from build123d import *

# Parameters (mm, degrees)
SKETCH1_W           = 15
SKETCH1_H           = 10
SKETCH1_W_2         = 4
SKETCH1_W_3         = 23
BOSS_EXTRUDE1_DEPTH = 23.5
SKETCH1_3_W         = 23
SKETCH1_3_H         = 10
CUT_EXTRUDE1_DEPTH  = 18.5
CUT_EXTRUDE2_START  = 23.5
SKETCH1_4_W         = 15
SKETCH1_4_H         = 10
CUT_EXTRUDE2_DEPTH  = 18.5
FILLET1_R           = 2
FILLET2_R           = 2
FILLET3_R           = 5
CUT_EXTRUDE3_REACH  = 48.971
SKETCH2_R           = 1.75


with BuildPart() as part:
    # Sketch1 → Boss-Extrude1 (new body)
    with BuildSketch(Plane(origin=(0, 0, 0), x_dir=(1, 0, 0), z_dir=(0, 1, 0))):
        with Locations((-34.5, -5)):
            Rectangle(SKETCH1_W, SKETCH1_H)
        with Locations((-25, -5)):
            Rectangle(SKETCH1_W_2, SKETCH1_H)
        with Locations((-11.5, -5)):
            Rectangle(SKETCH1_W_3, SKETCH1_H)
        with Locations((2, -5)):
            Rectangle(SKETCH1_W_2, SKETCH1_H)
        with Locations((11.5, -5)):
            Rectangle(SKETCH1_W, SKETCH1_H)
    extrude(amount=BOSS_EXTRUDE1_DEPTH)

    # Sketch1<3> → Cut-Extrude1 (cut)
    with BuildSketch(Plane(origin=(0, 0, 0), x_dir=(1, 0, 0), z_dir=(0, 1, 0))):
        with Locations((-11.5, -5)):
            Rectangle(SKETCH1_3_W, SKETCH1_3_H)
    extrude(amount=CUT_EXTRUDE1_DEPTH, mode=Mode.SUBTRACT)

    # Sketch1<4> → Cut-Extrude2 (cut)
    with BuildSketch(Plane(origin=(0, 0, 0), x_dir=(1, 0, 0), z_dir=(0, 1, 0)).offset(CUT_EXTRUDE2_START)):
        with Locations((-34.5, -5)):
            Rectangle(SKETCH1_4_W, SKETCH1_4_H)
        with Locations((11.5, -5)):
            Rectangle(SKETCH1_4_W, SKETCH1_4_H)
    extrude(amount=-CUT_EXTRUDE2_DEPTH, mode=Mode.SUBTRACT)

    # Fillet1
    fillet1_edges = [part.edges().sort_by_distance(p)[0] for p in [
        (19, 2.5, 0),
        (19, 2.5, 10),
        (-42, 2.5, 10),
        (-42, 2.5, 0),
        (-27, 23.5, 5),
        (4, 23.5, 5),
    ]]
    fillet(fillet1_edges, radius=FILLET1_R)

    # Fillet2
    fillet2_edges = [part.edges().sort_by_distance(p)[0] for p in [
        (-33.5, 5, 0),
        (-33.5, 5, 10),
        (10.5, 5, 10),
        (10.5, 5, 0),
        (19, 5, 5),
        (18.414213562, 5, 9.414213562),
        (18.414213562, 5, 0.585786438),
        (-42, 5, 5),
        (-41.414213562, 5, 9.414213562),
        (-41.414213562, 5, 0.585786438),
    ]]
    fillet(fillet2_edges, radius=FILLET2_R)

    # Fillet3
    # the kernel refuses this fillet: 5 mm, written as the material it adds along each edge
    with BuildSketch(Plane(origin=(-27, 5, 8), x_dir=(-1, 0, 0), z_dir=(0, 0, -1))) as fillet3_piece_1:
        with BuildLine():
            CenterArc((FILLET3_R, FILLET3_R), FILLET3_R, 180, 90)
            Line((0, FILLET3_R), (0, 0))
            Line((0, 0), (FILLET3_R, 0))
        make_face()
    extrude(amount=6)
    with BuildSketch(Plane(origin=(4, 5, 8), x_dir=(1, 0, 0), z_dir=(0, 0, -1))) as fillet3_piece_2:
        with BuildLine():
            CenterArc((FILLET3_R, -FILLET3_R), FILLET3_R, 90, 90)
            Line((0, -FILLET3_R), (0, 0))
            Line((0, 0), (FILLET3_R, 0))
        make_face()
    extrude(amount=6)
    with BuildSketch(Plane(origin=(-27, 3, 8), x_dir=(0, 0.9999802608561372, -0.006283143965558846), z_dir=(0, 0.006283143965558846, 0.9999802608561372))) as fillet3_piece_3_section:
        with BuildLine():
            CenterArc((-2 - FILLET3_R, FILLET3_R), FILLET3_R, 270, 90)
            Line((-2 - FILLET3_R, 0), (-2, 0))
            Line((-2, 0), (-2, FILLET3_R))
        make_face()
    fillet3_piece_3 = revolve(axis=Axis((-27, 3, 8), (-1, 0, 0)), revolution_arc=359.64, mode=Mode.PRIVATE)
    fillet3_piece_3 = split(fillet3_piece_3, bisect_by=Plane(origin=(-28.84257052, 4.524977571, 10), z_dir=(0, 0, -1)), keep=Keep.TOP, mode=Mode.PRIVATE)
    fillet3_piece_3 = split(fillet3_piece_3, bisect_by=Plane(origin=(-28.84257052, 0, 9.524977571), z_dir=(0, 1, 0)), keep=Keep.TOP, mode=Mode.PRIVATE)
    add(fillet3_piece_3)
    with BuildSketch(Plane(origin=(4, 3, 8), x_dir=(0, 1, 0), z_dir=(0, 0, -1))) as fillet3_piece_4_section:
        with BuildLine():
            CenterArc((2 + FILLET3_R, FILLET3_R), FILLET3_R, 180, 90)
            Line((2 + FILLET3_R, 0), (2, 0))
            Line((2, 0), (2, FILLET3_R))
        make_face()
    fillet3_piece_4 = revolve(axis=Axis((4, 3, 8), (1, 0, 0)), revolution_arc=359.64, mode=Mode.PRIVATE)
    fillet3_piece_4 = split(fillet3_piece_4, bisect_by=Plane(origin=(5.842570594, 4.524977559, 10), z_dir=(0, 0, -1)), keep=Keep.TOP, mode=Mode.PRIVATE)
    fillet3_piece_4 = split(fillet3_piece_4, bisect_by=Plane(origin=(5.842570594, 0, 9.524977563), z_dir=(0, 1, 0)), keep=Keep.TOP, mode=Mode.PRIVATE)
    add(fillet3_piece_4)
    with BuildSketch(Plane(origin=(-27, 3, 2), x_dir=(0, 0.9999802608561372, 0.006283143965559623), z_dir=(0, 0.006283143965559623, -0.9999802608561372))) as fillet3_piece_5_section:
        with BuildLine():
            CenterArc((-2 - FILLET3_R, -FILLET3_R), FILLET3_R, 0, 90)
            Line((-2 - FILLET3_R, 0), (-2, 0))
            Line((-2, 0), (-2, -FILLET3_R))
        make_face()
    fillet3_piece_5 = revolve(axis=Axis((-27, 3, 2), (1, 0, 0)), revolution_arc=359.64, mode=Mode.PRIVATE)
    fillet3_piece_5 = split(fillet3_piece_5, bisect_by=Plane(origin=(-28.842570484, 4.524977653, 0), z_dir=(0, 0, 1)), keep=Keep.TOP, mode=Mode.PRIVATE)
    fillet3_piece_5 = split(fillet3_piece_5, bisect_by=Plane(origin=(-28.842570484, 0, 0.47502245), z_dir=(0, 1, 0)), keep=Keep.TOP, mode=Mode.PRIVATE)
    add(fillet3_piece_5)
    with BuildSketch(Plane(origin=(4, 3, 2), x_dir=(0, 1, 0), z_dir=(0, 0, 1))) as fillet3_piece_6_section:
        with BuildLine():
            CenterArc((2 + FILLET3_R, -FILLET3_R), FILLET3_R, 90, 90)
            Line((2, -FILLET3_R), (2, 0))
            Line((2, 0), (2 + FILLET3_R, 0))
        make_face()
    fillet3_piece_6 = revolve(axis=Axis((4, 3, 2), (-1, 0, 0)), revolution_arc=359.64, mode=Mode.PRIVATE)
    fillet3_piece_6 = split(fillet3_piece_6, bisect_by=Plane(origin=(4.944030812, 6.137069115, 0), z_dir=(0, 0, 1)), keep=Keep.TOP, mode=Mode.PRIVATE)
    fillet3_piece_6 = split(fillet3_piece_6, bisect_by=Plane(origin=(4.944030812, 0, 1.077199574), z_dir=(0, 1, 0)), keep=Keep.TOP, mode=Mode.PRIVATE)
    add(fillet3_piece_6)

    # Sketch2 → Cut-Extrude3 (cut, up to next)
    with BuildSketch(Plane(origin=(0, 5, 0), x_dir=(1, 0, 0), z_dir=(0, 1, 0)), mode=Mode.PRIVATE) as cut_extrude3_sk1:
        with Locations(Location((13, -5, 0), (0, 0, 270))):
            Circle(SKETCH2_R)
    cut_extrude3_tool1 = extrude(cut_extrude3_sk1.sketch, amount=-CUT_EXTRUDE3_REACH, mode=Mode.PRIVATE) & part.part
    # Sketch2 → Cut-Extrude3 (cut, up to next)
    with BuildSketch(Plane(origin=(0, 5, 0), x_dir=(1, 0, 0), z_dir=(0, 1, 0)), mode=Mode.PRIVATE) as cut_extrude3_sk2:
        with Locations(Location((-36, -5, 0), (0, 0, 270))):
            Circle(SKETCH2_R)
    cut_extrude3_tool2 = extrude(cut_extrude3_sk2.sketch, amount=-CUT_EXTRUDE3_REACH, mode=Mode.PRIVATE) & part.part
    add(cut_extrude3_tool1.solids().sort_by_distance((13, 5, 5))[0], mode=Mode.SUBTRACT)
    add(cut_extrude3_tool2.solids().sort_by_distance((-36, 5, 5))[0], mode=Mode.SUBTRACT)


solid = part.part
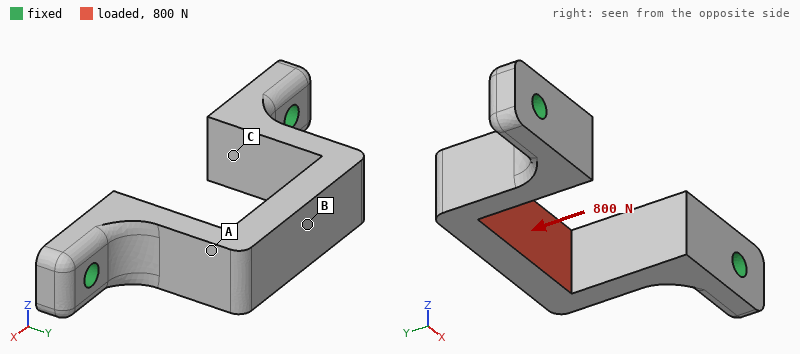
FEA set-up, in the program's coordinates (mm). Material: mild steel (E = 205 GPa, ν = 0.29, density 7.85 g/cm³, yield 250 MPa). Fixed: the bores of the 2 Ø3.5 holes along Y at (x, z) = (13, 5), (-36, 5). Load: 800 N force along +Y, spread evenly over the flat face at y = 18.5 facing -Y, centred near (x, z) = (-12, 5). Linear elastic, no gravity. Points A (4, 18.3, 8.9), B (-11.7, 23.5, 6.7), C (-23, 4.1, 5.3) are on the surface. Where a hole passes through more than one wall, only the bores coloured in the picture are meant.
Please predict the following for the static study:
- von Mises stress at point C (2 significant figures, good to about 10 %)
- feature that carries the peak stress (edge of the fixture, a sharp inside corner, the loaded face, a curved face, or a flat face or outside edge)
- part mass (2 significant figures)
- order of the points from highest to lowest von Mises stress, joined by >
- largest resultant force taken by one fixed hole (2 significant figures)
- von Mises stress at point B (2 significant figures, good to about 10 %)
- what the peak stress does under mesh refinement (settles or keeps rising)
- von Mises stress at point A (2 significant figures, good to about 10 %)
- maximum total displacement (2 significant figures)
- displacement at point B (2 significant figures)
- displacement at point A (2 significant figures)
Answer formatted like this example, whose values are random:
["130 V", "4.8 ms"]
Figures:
["9.3 MPa", "edge of the fixture", "35 g", "B > A > C", "450 N", "37 MPa", "keeps rising", "25 MPa", "8.0 µm", "7.7 µm", "3.2 µm"]
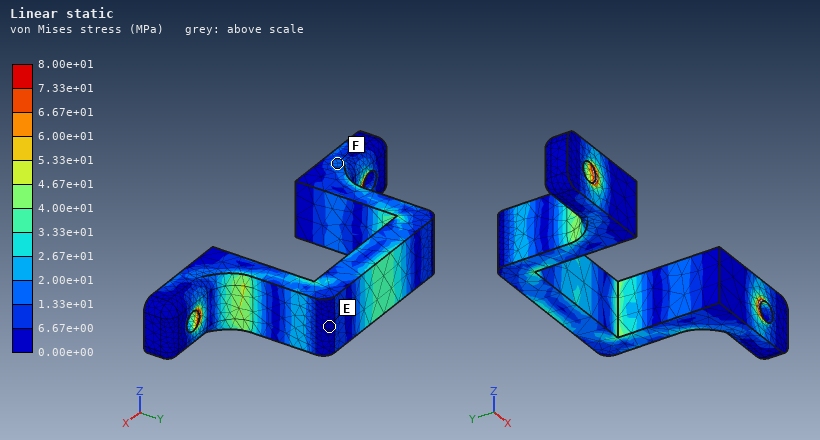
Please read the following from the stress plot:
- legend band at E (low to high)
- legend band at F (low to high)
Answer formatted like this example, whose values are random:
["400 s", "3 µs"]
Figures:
["0.00e+00 to 6.67e+00 MPa", "1.33e+01 to 2.00e+01 MPa"]
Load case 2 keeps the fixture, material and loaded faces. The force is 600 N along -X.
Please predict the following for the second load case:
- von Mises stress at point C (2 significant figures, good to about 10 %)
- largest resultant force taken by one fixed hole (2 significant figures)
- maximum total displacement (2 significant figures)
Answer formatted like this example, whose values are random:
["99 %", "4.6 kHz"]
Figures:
["20 MPa", "330 N", "17 µm"]
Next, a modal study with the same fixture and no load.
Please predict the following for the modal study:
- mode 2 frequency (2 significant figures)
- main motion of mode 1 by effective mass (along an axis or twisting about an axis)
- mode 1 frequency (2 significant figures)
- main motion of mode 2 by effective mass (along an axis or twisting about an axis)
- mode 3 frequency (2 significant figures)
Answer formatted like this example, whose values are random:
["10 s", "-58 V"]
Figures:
["7800 Hz", "along Z", "4900 Hz", "along X", "10 kHz"]
